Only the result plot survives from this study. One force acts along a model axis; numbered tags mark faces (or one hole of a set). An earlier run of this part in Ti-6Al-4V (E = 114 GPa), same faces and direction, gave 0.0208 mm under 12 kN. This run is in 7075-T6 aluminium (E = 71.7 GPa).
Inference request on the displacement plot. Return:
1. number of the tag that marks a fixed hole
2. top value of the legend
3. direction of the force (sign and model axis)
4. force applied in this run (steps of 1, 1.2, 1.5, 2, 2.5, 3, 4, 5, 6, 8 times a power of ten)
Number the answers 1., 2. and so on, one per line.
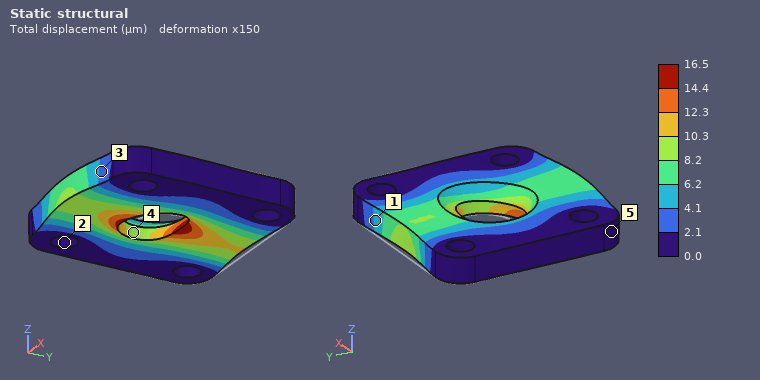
1. 2
2. 16.5 µm
3. -Y
4. 6 kN
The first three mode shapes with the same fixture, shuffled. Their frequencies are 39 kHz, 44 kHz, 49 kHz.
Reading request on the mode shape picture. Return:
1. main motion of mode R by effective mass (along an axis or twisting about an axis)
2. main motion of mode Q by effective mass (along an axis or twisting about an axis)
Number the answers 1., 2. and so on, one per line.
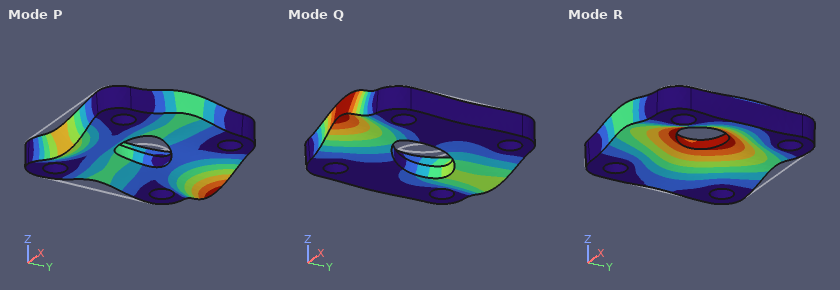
1. along Z
2. twisting about X
